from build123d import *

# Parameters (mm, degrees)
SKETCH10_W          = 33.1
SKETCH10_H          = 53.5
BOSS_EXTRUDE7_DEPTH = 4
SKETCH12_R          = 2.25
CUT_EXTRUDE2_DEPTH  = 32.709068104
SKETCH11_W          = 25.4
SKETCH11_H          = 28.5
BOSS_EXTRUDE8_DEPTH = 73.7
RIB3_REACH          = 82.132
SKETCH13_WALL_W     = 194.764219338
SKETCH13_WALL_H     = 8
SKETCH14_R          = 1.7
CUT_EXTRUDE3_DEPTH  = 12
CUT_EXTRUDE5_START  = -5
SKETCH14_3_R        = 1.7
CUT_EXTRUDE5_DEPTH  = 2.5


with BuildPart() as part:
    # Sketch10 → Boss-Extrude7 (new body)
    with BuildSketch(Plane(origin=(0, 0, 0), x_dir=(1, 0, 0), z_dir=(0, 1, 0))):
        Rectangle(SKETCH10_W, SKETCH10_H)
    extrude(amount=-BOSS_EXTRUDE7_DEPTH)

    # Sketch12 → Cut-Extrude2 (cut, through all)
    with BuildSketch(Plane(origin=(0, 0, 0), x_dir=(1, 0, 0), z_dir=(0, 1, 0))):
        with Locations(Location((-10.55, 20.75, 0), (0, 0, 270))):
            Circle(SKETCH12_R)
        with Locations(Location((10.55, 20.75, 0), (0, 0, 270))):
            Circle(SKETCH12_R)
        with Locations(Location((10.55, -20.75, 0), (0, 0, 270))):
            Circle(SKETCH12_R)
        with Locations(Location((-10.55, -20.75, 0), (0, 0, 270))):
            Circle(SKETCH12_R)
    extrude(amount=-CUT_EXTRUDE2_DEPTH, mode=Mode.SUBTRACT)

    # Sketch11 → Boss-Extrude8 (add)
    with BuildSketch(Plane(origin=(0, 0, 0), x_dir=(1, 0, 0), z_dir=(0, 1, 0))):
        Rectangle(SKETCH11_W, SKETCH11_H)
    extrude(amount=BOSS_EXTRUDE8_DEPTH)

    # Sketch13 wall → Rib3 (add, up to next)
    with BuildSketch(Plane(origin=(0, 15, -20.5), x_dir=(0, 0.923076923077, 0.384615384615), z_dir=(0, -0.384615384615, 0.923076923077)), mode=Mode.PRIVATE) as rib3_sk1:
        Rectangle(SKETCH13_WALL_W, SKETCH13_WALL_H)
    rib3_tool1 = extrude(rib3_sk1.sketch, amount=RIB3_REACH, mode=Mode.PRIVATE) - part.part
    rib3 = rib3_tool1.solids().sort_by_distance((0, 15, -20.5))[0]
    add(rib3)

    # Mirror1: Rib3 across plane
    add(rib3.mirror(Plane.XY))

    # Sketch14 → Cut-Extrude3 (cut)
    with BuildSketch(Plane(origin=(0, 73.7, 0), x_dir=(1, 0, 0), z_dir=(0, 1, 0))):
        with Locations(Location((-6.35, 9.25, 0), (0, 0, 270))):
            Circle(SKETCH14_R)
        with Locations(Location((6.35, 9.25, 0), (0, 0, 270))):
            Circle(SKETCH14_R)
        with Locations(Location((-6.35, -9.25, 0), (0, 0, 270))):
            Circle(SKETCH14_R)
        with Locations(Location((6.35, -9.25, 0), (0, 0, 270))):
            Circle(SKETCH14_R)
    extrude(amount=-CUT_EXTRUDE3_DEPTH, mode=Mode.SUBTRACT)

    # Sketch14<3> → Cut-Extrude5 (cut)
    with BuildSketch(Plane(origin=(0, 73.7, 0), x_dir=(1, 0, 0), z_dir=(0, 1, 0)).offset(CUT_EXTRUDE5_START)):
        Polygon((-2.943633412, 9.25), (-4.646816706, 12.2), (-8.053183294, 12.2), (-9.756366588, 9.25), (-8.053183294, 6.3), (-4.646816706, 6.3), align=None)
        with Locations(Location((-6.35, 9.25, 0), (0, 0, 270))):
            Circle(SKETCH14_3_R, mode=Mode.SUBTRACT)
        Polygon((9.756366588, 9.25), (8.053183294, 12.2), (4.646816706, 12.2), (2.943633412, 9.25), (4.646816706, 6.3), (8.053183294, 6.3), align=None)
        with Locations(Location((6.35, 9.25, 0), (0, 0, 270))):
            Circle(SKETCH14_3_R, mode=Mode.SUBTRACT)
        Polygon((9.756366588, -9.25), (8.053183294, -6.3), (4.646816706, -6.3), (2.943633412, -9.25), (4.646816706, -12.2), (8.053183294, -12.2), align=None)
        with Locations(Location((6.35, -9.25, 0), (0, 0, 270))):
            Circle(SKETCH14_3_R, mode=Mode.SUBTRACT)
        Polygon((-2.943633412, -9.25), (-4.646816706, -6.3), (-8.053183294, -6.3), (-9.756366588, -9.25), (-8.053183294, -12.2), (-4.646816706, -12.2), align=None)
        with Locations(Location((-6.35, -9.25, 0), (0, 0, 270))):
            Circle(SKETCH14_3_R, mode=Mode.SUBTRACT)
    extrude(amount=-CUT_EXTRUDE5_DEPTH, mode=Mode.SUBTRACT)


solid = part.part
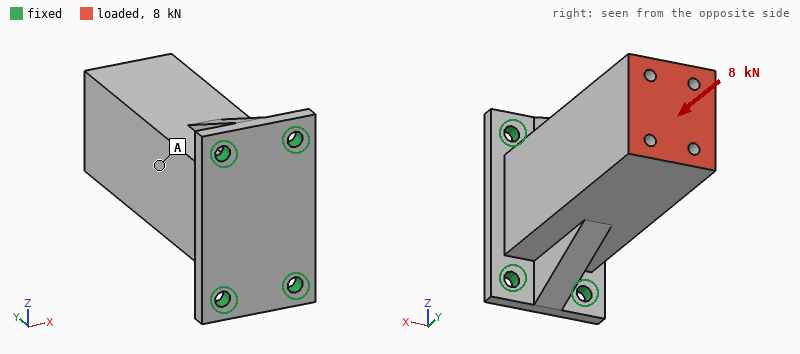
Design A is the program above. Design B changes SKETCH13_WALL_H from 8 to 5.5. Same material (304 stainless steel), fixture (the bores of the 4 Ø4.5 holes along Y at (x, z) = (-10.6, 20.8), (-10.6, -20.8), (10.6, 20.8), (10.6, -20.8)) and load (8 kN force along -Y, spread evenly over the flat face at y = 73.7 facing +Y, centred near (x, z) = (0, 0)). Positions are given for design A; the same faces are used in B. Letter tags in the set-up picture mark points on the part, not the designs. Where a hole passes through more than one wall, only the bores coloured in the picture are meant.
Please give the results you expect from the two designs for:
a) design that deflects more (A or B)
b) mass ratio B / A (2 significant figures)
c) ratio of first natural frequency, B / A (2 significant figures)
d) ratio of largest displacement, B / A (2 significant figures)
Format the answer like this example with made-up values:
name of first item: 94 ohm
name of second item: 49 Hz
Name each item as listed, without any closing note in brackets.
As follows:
design that deflects more: B
mass ratio B / A: 0.99
ratio of first natural frequency, B / A: 0.96
ratio of largest displacement, B / A: 1.1
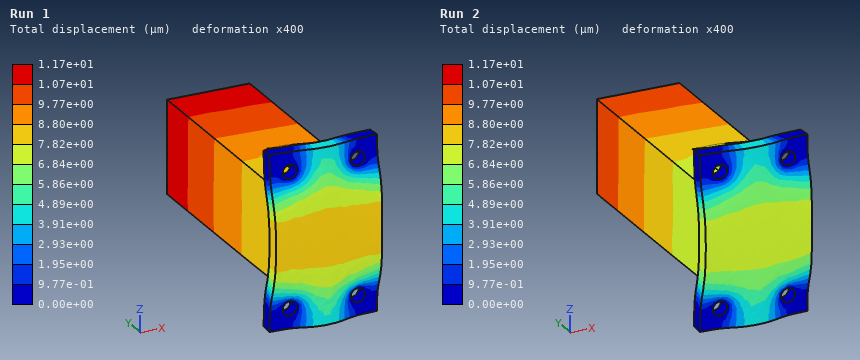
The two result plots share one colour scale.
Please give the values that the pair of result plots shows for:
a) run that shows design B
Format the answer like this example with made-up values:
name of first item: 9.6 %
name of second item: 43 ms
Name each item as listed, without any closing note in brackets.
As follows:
run that shows design B: Run 1
